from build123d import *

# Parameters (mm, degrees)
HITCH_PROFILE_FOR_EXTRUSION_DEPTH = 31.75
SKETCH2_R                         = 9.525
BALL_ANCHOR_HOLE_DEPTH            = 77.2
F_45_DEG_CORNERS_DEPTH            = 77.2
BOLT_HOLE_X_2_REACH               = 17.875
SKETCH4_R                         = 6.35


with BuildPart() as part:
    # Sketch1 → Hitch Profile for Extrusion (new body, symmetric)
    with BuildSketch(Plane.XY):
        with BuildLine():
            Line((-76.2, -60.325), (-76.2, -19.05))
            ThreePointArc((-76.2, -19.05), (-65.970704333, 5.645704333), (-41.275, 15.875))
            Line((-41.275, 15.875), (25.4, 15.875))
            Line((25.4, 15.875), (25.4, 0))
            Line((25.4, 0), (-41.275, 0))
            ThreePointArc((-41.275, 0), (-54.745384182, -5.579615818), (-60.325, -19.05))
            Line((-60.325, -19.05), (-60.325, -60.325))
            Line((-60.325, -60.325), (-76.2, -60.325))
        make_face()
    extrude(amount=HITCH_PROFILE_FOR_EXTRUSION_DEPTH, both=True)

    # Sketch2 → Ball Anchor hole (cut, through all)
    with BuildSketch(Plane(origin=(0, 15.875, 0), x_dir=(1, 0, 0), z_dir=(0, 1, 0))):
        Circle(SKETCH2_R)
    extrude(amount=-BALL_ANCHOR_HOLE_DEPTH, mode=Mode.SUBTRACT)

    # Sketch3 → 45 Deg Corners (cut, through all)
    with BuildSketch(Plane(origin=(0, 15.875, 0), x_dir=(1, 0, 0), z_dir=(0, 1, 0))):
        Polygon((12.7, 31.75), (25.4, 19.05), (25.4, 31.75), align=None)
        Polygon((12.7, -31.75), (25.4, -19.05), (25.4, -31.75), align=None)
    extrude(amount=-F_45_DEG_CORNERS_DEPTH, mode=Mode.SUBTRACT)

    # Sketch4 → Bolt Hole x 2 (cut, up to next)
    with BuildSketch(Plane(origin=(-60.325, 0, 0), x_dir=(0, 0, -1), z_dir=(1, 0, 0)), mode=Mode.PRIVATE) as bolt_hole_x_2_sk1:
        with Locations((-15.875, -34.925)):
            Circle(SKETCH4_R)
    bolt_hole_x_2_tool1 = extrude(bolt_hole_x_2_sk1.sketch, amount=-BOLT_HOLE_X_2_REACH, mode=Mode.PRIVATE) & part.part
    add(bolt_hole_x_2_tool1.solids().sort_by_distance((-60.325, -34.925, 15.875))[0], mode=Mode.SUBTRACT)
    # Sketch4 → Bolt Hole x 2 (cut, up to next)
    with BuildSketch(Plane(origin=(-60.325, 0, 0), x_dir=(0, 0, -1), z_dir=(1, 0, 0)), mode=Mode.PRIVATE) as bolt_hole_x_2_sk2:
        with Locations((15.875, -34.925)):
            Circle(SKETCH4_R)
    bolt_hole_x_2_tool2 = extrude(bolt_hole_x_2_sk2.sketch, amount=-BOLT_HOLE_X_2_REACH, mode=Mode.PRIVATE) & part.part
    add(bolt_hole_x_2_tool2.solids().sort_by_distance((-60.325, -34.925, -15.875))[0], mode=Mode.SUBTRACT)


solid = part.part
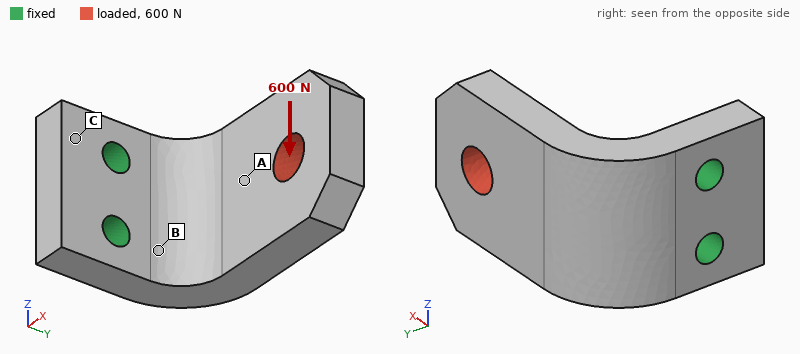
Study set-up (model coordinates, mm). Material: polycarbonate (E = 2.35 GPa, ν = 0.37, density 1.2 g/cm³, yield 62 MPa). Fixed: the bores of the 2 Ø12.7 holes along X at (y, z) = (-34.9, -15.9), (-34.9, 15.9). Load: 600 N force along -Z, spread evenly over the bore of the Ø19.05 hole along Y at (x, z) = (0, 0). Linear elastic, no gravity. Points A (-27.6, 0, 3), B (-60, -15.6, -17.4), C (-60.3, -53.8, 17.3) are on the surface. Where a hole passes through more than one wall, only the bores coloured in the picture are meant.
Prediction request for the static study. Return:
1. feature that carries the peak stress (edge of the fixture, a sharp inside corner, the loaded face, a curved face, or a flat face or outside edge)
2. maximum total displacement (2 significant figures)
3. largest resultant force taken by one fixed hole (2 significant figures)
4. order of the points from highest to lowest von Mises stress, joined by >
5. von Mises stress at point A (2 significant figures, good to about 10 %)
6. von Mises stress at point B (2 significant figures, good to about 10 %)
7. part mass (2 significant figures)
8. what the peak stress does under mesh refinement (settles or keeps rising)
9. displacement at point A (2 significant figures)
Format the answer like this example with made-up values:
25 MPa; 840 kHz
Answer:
edge of the fixture; 1.3 mm; 1.1 kN; B > A > C; 2.9 MPa; 9.2 MPa; 170 g; keeps rising; 0.54 mm
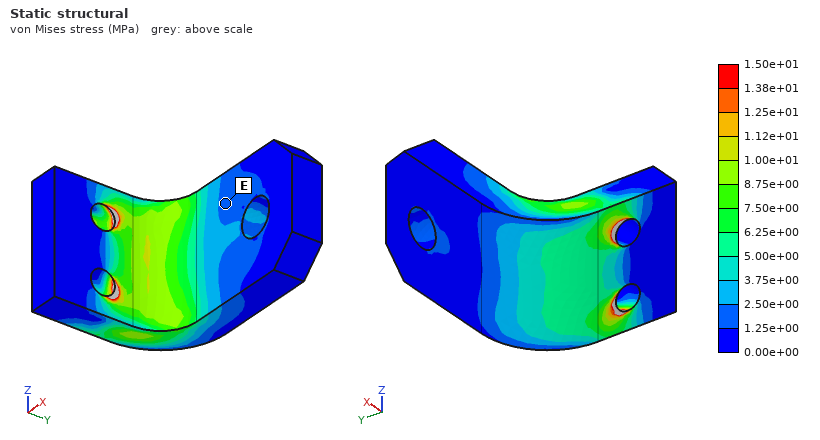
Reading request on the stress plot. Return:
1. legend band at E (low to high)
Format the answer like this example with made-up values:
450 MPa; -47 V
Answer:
1.25e+00 to 2.50e+00 MPa
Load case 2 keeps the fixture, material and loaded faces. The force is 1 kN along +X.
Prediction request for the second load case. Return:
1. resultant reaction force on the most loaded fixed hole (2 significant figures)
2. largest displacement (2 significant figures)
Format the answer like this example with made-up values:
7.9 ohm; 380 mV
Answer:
500 N; 1.7 mm
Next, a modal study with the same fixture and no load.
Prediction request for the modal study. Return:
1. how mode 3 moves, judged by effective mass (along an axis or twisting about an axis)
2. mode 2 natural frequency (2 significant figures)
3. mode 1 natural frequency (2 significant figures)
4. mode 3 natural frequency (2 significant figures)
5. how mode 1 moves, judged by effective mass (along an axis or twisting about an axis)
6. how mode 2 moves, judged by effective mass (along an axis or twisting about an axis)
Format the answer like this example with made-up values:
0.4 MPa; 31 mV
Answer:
along X; 500 Hz; 290 Hz; 1100 Hz; along Y; along Z
